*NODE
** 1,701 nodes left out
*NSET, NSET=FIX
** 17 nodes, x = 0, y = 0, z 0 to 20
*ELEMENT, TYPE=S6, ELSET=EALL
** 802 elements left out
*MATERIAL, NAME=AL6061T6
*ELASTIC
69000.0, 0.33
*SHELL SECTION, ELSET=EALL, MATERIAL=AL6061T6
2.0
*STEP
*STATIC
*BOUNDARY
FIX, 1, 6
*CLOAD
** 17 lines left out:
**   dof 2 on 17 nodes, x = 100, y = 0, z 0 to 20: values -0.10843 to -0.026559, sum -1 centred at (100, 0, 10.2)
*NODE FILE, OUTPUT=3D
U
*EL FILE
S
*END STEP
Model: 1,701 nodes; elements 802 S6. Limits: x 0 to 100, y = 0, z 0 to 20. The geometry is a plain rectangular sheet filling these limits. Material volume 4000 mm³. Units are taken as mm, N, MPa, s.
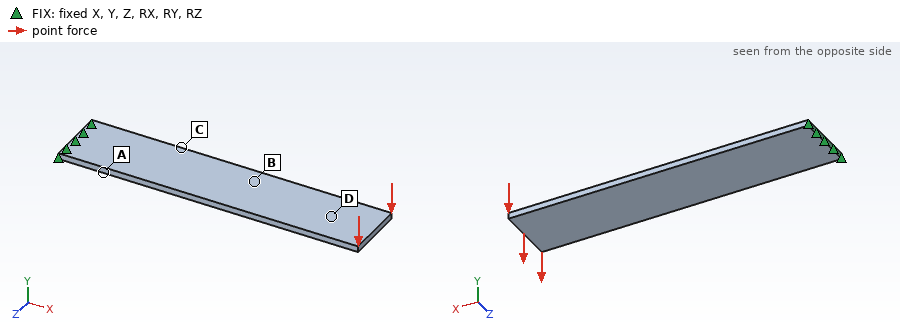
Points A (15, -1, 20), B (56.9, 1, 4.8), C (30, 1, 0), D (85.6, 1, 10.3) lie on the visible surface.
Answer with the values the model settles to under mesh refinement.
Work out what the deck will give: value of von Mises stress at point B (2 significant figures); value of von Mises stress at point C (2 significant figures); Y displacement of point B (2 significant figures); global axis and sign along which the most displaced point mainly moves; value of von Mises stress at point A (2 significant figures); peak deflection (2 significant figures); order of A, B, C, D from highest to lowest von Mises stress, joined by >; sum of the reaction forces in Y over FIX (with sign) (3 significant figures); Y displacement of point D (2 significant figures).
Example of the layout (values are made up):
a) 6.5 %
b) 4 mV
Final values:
a) 3.2 MPa
b) 5.3 MPa
c) -0.14 mm
d) -Y
e) 6.5 MPa
f) 0.35 mm
g) A > C > B > D
h) 1.00 N
i) -0.28 mm
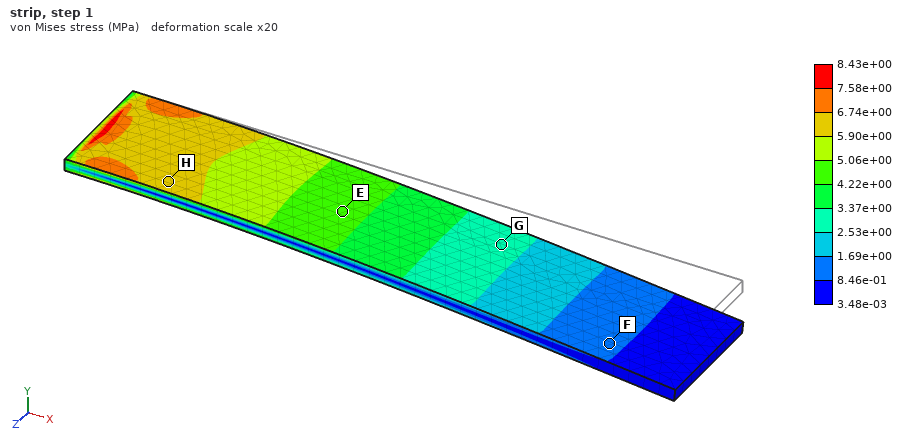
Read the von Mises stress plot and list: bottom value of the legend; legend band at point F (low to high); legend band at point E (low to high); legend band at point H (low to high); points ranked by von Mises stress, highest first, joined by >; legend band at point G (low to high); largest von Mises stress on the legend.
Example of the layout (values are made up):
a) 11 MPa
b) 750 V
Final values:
a) 3.48e-03 MPa
b) 8.46e-01 to 1.69e+00 MPa
c) 4.22e+00 to 5.06e+00 MPa
d) 5.90e+00 to 6.74e+00 MPa
e) H > E > G > F
f) 2.53e+00 to 3.37e+00 MPa
g) 8.43e+00 MPa
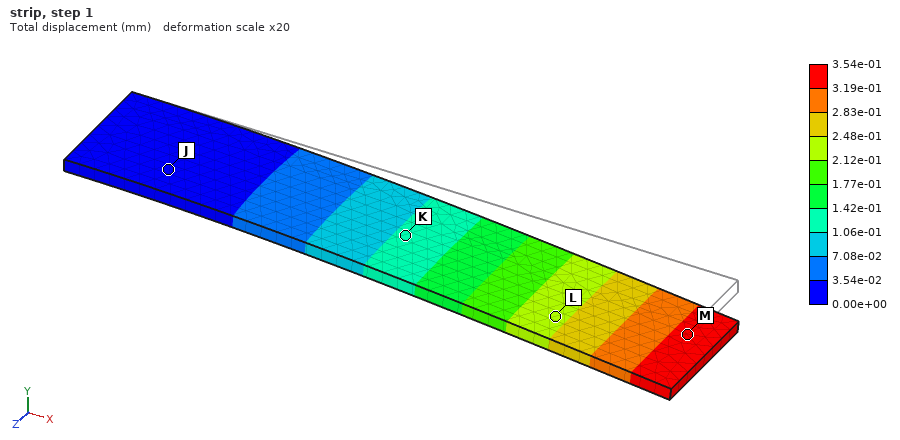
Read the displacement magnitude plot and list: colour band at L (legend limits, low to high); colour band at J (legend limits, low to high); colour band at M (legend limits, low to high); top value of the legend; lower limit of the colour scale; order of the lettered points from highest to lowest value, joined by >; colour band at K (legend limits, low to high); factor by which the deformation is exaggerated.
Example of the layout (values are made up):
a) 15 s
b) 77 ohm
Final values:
a) 2.12e-01 to 2.48e-01 mm
b) 0.00e+00 to 3.54e-02 mm
c) 3.19e-01 to 3.54e-01 mm
d) 3.54e-01 mm
e) 0.00e+00 mm
f) M > L > K > J
g) 1.06e-01 to 1.42e-01 mm
h) 20
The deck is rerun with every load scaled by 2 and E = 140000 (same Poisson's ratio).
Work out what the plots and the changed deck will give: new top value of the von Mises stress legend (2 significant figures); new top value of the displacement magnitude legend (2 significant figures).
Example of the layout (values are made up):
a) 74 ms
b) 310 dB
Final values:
a) 17 MPa
b) 0.35 mm
